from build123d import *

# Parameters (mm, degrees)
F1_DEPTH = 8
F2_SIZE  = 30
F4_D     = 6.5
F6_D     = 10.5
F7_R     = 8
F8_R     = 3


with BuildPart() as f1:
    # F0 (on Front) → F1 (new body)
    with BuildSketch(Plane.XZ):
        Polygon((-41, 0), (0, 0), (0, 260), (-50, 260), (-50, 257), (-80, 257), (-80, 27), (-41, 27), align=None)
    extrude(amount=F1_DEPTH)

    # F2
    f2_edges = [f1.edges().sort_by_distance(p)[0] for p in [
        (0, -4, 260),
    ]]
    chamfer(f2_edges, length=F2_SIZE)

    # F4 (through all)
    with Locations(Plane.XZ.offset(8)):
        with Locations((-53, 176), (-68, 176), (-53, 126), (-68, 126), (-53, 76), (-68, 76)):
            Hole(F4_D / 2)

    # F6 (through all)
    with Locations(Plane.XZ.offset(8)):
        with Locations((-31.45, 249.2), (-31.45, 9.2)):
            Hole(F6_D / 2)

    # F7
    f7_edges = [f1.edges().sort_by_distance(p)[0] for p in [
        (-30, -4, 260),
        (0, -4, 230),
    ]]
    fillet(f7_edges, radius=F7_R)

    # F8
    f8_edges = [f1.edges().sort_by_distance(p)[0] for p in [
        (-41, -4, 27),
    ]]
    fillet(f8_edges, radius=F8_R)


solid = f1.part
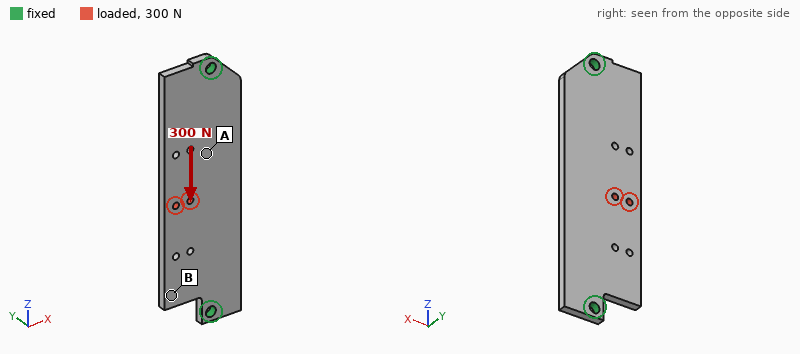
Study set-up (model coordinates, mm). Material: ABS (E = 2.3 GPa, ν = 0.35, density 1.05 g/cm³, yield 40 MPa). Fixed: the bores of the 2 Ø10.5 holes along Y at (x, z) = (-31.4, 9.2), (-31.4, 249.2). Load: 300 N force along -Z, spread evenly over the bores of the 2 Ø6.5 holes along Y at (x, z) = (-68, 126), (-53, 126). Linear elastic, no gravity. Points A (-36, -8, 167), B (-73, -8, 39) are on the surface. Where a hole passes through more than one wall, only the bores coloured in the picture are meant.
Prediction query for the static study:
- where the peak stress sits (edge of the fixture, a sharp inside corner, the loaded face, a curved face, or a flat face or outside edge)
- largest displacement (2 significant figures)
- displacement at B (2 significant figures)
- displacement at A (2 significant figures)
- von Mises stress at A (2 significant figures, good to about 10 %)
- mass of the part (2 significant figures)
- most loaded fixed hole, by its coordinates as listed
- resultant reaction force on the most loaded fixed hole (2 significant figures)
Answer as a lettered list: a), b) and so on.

a) a curved face
b) 28 µm
c) 19 µm
d) 15 µm
e) 0.30 MPa
f) 160 g
g) (-31.4, 249.2)
h) 170 N
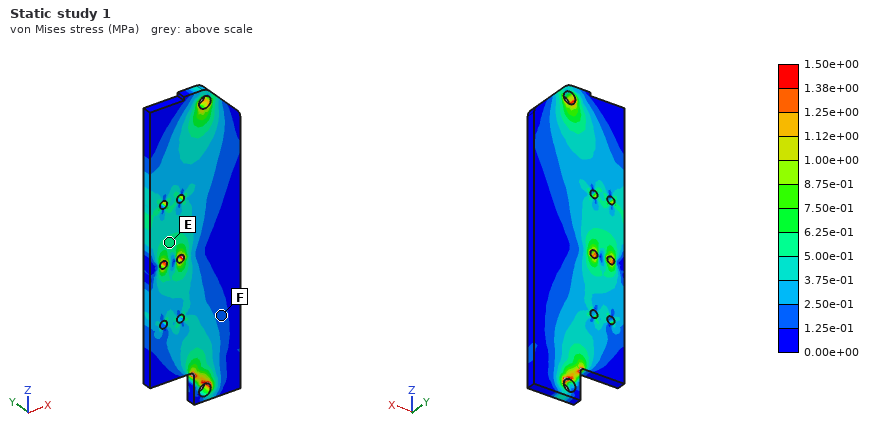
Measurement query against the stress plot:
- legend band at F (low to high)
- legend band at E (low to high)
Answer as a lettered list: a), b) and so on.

a) 1.25e-01 to 2.50e-01 MPa
b) 5.00e-01 to 6.25e-01 MPa
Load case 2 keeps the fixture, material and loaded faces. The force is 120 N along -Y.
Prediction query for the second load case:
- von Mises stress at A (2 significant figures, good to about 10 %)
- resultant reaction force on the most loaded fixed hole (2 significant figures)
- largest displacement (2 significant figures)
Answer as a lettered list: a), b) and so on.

a) 2.2 MPa
b) 61 N
c) 2.3 mm
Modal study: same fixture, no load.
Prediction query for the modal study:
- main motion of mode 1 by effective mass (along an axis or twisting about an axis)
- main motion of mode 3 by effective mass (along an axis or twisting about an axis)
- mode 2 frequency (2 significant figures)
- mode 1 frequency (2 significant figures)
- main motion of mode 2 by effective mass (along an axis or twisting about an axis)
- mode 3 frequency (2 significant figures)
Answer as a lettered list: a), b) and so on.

a) along Y
b) twisting about X
c) 310 Hz
d) 180 Hz
e) twisting about Z
f) 480 Hz
